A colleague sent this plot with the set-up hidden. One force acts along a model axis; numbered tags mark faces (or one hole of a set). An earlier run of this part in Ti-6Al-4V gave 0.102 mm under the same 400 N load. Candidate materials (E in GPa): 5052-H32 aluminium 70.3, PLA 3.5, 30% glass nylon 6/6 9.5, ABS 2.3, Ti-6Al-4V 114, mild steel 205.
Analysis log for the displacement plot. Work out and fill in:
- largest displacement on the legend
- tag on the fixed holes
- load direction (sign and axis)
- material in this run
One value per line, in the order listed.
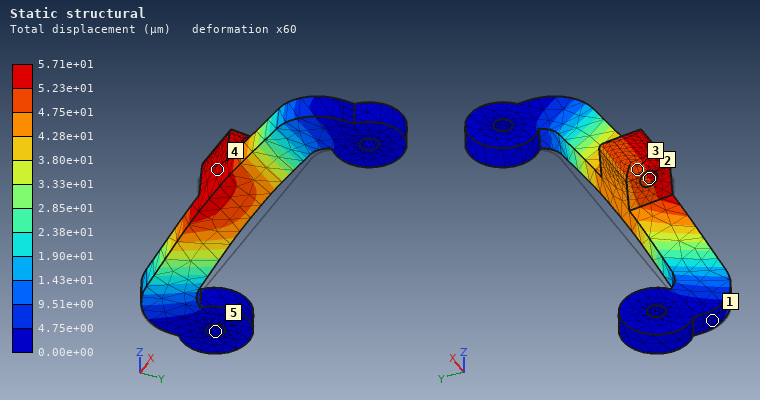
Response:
5.71e+01 µm
5
+Z
mild steel
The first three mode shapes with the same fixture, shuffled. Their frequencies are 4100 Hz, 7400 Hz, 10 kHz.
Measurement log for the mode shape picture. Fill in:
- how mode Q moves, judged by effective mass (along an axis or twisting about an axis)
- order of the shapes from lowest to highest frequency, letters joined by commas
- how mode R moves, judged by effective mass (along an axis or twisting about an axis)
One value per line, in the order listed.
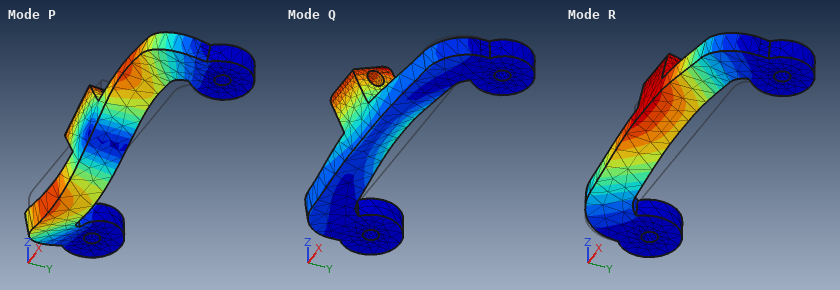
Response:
along Y
R, Q, P
along Z
